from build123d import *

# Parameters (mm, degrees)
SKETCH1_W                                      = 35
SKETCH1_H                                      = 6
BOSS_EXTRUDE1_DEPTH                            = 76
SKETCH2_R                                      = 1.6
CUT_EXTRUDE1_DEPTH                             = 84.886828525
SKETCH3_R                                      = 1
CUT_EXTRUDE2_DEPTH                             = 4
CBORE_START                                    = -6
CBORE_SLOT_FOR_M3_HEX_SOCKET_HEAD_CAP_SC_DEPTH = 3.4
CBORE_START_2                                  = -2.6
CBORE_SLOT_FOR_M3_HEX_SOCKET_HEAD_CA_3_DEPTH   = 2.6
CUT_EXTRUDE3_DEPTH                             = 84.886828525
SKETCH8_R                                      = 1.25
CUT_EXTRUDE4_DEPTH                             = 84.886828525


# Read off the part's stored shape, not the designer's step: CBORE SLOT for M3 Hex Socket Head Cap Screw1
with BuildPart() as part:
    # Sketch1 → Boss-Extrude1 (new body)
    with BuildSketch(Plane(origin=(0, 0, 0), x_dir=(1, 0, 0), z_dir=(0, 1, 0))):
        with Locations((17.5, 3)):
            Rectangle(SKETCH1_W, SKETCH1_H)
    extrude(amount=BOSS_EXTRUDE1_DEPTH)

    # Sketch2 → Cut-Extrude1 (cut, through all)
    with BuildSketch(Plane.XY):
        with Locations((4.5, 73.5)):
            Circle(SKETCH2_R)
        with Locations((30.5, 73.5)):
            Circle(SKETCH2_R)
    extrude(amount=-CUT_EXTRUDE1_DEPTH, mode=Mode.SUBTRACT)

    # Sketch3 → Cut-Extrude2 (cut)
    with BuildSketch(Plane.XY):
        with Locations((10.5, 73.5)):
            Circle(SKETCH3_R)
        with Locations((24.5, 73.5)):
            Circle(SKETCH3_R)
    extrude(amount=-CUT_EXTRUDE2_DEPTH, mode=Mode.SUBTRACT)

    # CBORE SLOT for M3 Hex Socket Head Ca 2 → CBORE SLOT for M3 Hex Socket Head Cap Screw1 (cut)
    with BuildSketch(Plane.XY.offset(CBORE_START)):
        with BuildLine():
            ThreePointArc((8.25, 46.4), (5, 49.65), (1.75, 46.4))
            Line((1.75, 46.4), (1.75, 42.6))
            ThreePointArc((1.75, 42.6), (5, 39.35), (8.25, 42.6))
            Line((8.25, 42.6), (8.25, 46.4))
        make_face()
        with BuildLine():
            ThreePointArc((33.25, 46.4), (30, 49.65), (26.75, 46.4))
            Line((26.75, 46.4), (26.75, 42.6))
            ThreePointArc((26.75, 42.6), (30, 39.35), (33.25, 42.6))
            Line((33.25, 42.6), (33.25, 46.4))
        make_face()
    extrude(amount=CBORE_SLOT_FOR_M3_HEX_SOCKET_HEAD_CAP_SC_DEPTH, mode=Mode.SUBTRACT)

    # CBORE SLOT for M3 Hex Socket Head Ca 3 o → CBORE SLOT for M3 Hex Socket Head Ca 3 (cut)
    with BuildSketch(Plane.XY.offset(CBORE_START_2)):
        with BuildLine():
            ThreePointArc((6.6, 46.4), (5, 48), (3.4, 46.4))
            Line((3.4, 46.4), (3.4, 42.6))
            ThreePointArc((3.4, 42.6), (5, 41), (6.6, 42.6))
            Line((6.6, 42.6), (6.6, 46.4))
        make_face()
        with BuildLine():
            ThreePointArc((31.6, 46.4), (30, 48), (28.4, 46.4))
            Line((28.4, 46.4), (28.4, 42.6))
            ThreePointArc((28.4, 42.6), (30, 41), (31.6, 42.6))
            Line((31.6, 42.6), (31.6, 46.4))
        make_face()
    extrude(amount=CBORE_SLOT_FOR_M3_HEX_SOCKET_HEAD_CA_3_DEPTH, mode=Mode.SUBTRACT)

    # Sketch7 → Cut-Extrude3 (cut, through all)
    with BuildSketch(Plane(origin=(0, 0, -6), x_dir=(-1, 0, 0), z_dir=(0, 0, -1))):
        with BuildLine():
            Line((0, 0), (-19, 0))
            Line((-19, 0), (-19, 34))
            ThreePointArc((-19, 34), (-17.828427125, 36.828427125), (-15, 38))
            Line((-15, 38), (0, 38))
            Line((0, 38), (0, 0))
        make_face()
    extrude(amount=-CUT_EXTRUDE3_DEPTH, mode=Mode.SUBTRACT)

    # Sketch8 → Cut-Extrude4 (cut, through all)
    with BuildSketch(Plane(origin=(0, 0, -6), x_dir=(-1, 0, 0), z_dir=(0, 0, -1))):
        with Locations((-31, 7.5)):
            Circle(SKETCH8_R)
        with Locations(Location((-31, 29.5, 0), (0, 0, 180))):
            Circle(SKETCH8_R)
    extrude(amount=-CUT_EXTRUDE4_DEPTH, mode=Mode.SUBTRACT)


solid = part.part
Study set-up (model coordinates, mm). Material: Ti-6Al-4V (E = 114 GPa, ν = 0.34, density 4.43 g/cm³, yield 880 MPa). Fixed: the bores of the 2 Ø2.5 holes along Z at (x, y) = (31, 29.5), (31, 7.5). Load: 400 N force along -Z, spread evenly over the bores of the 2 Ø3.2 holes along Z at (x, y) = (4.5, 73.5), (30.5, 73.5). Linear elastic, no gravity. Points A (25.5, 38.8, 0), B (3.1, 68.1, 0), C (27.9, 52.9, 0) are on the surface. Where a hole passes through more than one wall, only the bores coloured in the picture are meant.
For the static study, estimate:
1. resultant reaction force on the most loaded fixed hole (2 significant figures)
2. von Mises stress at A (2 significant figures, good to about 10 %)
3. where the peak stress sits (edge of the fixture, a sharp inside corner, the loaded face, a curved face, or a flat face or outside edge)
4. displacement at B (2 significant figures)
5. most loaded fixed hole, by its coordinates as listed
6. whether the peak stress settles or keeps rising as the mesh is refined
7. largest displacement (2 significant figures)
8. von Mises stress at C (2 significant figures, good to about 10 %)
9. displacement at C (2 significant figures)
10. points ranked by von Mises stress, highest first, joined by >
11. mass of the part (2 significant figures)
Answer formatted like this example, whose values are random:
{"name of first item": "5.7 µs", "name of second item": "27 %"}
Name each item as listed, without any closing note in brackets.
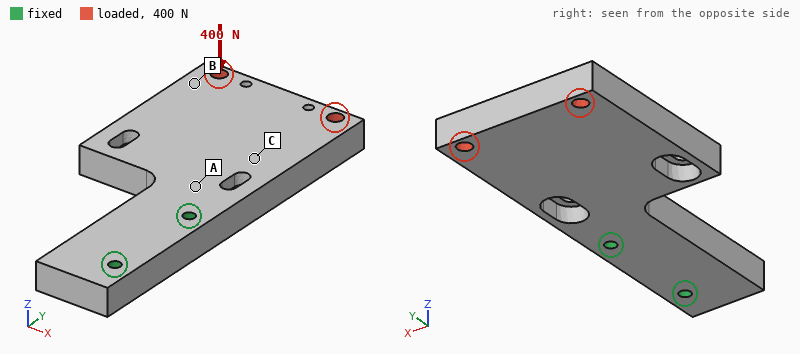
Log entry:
{"resultant reaction force on the most loaded fixed hole": "730 N", "von Mises stress at A": "150 MPa", "where the peak stress sits": "edge of the fixture", "displacement at B": "0.39 mm", "most loaded fixed hole, by its coordinates as listed": "(31, 29.5)", "whether the peak stress settles or keeps rising as the mesh is refined": "keeps rising", "largest displacement": "0.49 mm", "von Mises stress at C": "49 MPa", "displacement at C": "0.15 mm", "points ranked by von Mises stress, highest first, joined by >": "A > C > B", "mass of the part": "49 g"}
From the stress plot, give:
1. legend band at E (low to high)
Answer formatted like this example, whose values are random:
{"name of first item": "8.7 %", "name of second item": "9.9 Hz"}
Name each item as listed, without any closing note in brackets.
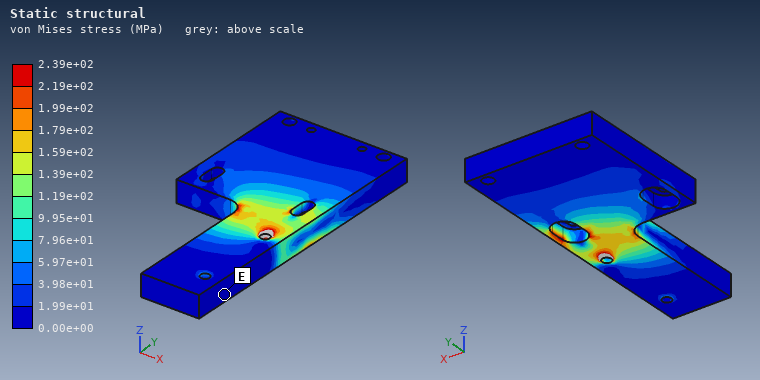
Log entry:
{"legend band at E": "0.00e+00 to 1.99e+01 MPa"}
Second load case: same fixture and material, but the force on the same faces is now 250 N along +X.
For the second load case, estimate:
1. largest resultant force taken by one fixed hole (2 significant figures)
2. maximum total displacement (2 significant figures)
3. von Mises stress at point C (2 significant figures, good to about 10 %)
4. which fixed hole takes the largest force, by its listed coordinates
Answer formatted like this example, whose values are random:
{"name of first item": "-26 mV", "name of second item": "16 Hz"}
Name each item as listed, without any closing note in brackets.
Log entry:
{"largest resultant force taken by one fixed hole": "810 N", "maximum total displacement": "56 µm", "von Mises stress at point C": "7.1 MPa", "which fixed hole takes the largest force, by its listed coordinates": "(31, 29.5)"}
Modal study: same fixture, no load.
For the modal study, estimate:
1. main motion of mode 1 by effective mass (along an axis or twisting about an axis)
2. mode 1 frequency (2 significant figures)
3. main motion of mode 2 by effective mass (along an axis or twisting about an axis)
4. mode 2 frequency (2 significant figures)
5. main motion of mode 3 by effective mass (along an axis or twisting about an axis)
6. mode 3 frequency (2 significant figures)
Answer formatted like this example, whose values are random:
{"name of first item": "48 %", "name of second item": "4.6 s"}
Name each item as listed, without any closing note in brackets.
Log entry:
{"main motion of mode 1 by effective mass": "along Z", "mode 1 frequency": "1300 Hz", "main motion of mode 2 by effective mass": "along X", "mode 2 frequency": "2800 Hz", "main motion of mode 3 by effective mass": "twisting about Y", "mode 3 frequency": "3500 Hz"}
